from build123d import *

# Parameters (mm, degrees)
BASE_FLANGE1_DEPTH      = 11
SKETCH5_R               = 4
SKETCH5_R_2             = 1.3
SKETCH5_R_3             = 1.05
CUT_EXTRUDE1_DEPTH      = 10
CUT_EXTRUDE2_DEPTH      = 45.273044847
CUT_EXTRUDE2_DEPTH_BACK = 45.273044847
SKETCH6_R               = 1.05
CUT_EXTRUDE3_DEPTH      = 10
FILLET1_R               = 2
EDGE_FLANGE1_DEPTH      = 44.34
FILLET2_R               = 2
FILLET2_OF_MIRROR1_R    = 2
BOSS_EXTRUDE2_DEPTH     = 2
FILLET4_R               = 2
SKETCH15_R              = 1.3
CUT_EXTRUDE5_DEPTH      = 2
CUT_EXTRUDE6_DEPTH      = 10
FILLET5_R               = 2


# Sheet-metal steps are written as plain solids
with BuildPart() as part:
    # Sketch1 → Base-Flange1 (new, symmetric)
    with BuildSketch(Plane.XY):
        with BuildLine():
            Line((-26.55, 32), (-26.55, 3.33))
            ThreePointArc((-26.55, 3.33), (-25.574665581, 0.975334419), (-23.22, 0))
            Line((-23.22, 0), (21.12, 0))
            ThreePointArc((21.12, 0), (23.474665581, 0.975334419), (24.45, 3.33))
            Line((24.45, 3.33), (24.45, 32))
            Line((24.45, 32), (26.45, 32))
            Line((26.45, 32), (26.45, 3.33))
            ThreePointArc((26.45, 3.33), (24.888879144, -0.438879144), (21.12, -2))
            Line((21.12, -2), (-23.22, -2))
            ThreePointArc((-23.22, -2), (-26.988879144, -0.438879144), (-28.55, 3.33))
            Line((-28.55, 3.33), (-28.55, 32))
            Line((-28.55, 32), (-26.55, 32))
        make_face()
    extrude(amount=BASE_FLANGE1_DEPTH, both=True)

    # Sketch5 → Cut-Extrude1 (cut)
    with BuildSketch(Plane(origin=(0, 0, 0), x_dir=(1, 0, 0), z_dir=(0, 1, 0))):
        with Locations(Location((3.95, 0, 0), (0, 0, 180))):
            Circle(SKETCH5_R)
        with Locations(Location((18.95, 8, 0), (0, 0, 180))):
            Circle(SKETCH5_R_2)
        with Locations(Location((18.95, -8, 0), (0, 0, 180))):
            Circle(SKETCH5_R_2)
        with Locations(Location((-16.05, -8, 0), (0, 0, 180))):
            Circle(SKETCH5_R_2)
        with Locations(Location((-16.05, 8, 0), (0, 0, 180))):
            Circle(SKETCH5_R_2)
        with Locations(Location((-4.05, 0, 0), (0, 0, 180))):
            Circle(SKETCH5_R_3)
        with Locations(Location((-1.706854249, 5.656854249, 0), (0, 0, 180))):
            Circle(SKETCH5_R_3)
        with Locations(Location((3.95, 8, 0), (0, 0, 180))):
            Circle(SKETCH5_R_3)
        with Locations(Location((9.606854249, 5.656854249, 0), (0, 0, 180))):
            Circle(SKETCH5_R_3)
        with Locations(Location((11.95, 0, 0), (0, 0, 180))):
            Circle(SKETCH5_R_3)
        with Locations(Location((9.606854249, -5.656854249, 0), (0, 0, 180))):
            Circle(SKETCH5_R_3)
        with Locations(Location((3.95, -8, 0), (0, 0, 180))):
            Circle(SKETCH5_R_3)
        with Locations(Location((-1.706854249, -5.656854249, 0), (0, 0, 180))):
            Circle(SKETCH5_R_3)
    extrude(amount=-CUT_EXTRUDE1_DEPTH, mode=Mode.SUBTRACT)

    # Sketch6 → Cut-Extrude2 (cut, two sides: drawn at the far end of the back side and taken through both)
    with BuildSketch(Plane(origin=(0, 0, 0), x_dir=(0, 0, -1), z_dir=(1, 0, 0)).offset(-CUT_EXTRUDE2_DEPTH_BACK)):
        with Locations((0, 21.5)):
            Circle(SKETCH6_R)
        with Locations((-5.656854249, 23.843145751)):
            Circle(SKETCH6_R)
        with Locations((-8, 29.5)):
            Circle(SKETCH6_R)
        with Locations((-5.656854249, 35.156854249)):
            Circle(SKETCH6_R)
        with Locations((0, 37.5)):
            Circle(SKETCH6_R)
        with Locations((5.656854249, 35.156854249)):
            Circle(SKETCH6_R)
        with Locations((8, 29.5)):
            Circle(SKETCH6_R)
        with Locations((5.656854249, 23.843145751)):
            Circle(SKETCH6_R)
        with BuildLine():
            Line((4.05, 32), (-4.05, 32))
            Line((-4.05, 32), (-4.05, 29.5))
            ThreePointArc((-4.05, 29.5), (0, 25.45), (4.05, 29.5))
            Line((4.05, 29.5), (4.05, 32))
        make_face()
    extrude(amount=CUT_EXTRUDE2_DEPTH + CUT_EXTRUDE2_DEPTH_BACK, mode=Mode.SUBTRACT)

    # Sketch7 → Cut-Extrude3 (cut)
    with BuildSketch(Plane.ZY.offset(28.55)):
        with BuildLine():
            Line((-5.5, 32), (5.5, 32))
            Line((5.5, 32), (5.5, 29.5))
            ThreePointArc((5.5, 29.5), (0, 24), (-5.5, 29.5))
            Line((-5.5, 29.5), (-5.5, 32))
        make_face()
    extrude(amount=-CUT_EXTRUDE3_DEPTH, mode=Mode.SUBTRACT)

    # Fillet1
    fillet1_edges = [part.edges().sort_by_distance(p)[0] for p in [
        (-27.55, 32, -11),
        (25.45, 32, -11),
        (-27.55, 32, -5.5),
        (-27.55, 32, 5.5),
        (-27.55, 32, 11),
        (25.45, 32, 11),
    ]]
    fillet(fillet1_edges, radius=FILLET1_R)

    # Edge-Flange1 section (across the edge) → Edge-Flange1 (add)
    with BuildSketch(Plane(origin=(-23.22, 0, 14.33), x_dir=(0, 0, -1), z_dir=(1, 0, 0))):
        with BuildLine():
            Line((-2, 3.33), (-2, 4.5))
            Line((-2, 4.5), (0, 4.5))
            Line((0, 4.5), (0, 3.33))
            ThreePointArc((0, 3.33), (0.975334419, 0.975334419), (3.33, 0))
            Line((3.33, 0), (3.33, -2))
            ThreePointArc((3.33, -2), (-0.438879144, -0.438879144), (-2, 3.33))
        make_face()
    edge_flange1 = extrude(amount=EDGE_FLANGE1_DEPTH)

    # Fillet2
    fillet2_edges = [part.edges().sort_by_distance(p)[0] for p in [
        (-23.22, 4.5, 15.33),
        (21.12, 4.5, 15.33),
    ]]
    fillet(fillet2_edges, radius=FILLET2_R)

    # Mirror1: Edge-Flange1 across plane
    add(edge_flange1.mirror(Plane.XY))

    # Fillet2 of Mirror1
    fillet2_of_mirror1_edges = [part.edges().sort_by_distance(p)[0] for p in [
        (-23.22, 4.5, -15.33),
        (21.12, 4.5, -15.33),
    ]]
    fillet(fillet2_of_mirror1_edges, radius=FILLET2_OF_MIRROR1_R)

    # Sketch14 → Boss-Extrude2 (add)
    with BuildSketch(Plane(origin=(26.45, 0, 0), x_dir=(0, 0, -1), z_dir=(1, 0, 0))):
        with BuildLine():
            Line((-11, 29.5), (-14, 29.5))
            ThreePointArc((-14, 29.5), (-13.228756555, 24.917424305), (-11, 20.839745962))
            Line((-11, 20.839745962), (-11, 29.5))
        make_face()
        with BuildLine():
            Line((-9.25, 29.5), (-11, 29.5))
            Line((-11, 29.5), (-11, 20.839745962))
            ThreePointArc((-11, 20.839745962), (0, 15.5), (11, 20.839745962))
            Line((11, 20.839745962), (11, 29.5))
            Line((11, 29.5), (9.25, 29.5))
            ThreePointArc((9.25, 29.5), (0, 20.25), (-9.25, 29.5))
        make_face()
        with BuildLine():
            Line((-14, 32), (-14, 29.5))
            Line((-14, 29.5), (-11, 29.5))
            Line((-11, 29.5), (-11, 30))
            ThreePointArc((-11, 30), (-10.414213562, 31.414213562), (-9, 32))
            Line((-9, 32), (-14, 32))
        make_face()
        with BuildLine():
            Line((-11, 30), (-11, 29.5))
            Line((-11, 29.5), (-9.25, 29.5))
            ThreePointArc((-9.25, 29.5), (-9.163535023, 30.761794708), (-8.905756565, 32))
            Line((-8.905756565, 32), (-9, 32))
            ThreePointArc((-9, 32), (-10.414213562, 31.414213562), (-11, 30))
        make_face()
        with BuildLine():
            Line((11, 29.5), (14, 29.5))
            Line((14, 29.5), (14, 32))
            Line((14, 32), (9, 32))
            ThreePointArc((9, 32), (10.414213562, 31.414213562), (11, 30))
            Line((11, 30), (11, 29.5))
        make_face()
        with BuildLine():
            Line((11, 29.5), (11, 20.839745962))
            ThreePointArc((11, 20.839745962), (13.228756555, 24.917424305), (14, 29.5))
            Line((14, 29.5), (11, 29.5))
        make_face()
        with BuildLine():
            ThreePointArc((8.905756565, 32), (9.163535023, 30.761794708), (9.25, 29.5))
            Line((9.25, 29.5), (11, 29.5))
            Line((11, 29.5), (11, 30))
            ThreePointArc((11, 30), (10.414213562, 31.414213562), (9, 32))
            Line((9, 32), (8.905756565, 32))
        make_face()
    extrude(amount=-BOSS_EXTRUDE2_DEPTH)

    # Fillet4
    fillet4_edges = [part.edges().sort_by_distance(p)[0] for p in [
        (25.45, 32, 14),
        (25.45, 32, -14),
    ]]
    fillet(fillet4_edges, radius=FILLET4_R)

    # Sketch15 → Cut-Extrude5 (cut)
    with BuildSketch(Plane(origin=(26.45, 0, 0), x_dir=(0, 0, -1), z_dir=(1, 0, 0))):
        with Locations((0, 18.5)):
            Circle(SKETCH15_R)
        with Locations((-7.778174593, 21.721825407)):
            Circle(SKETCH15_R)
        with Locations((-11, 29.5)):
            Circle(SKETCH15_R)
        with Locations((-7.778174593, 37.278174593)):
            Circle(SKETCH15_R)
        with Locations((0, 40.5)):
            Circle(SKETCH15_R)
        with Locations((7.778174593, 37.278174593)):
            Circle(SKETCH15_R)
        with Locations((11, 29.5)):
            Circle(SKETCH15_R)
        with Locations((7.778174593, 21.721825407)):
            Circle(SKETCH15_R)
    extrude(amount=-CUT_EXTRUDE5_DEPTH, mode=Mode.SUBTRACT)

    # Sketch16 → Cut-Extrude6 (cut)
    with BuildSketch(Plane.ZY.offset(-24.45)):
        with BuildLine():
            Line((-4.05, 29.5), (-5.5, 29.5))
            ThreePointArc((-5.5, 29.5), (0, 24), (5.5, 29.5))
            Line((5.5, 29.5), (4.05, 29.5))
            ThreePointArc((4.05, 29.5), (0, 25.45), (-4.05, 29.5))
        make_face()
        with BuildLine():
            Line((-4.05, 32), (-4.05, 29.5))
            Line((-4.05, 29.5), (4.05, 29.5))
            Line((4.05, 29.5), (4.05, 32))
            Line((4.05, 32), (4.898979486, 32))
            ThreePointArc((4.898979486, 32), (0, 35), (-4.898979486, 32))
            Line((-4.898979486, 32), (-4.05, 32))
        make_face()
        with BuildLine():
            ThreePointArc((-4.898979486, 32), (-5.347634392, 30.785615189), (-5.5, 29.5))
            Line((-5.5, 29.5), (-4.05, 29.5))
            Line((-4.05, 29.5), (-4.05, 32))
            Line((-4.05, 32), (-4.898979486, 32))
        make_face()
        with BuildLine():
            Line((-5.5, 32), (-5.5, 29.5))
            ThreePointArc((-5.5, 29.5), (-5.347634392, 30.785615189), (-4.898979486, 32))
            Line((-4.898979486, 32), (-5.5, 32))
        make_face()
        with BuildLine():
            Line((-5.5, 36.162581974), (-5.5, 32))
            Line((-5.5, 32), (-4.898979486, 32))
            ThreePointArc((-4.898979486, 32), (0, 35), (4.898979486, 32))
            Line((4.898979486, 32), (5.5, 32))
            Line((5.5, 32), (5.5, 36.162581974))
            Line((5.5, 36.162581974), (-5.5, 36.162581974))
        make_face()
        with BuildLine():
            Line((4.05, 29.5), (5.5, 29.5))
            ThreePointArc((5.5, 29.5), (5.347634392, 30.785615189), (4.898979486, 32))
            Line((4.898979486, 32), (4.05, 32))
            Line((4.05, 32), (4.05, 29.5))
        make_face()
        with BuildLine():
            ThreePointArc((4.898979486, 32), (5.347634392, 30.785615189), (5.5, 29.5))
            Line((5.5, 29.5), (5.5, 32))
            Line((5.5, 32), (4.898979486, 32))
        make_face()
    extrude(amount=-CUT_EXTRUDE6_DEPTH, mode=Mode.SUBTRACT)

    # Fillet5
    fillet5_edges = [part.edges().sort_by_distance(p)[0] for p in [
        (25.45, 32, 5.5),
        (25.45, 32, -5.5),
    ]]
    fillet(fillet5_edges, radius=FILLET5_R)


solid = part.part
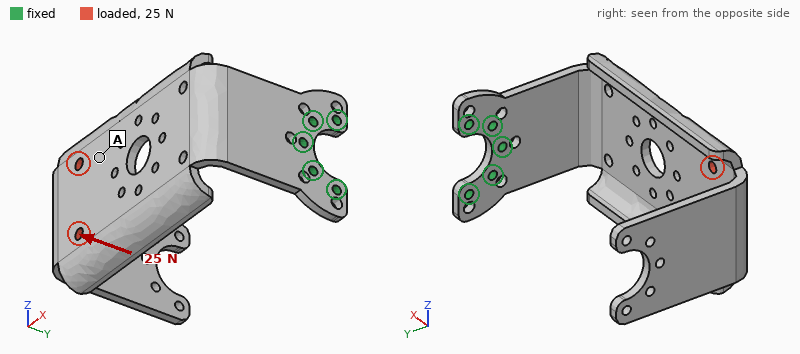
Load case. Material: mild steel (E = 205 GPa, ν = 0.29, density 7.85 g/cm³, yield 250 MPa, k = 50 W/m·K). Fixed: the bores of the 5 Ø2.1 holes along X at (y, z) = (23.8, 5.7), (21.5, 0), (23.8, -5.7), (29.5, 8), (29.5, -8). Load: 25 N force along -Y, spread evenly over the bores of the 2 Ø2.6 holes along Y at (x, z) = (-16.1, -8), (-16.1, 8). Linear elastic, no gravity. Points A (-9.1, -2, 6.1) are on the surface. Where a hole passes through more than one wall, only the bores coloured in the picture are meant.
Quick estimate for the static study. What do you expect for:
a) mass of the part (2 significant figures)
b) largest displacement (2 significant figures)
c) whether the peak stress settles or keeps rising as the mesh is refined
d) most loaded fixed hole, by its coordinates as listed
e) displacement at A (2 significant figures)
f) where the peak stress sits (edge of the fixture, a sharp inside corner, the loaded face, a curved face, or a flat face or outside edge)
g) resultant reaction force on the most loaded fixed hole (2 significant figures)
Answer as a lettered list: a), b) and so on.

a) 47 g
b) 0.61 mm
c) keeps rising
d) (21.5, 0)
e) 0.37 mm
f) a sharp inside corner
g) 82 N
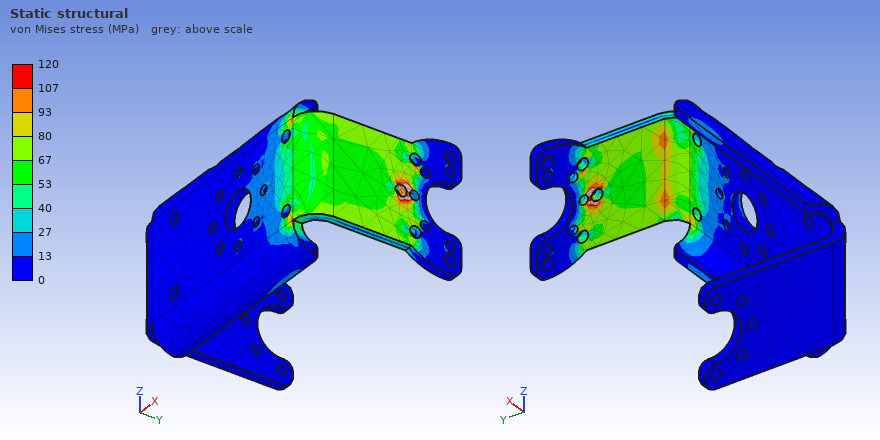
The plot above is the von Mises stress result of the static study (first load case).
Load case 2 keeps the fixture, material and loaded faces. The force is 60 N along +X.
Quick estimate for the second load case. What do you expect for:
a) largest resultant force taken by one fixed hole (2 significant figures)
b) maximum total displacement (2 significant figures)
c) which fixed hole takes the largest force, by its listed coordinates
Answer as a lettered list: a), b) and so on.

a) 120 N
b) 0.33 mm
c) (21.5, 0)
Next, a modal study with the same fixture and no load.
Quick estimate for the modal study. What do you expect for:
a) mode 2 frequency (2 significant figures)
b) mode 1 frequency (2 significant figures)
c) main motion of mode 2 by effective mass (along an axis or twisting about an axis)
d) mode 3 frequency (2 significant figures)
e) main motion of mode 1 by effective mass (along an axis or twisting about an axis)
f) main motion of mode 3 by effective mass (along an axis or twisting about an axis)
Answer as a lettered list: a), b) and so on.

a) 320 Hz
b) 210 Hz
c) along Z
d) 900 Hz
e) along Y
f) along X
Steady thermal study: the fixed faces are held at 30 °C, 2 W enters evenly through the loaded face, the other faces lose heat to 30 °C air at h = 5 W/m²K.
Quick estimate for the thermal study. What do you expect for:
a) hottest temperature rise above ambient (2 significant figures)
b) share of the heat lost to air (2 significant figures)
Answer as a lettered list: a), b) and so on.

a) 35 K
b) 39 %
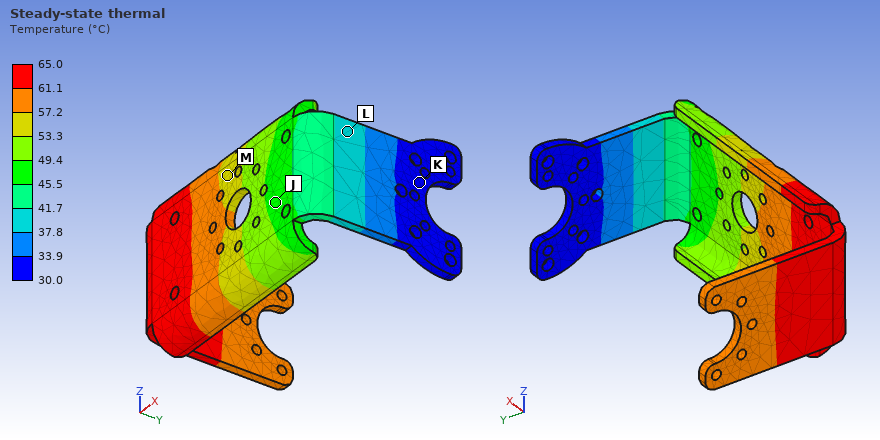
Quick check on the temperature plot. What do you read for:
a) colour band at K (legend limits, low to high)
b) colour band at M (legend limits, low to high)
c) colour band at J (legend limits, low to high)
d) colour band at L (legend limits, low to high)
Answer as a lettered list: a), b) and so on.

a) 30.0 to 33.9 °C
b) 53.3 to 57.2 °C
c) 45.5 to 49.4 °C
d) 37.8 to 41.7 °C
